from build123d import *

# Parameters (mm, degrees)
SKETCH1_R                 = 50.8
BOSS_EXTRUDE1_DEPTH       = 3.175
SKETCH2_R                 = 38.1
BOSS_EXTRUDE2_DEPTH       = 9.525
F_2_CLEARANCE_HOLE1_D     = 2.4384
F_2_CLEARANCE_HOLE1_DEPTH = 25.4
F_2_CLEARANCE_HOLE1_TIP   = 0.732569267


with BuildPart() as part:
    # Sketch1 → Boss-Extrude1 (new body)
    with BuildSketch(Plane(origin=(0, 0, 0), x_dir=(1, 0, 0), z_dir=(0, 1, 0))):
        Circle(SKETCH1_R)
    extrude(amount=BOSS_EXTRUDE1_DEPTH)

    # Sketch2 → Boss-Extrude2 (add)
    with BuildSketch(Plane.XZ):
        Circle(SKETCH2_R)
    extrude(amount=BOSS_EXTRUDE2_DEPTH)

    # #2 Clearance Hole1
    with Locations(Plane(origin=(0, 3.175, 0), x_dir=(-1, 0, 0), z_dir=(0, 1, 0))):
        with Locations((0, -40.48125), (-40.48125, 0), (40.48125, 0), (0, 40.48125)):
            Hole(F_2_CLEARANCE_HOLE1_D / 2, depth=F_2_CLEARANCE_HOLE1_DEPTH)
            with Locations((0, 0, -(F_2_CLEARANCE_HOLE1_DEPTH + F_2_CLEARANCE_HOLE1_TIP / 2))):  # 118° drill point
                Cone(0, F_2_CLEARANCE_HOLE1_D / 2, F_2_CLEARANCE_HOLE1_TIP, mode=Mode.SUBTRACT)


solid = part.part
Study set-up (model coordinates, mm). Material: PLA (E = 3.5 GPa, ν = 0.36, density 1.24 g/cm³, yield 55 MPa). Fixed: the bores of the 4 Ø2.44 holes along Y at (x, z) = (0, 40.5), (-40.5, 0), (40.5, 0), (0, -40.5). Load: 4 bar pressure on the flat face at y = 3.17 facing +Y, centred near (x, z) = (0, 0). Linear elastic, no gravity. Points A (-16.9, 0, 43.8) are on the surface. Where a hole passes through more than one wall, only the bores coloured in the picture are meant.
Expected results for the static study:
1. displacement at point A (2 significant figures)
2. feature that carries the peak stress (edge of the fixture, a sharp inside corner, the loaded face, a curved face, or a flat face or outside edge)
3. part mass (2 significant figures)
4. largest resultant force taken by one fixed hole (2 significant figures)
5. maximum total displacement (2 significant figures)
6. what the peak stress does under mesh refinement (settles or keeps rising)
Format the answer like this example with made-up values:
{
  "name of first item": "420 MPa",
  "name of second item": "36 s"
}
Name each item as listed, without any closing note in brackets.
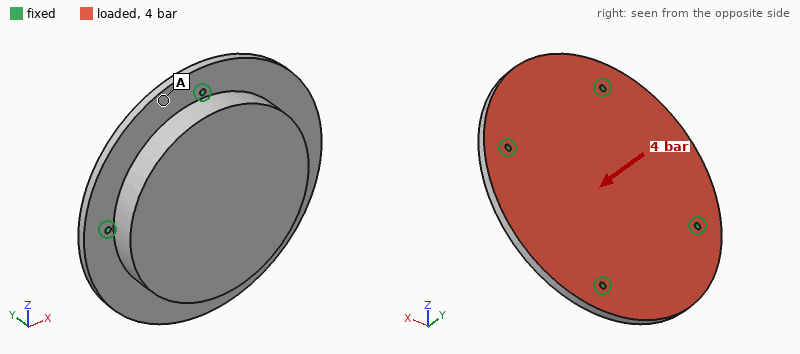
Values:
{
  "displacement at point A": "0.25 mm",
  "feature that carries the peak stress": "edge of the fixture",
  "part mass": "86 g",
  "largest resultant force taken by one fixed hole": "920 N",
  "maximum total displacement": "0.44 mm",
  "what the peak stress does under mesh refinement": "keeps rising"
}
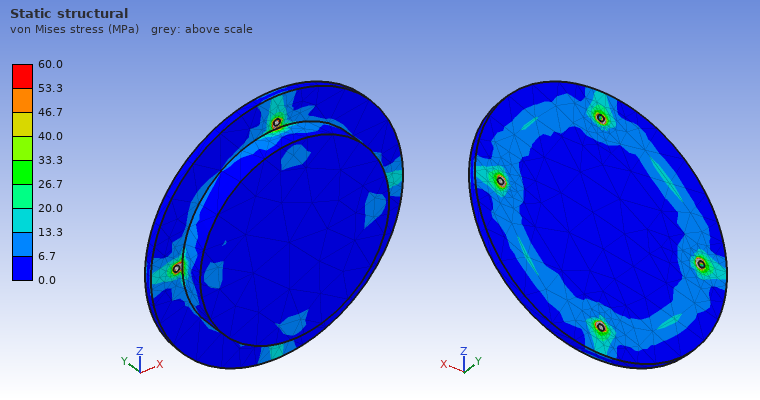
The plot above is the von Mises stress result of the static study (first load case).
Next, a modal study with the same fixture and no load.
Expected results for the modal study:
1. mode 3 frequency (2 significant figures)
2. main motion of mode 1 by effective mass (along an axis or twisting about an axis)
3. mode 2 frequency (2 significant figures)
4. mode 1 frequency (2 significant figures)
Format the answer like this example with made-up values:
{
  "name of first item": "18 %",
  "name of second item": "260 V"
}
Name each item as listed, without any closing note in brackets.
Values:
{
  "mode 3 frequency": "2500 Hz",
  "main motion of mode 1 by effective mass": "along Y",
  "mode 2 frequency": "2500 Hz",
  "mode 1 frequency": "2100 Hz"
}
